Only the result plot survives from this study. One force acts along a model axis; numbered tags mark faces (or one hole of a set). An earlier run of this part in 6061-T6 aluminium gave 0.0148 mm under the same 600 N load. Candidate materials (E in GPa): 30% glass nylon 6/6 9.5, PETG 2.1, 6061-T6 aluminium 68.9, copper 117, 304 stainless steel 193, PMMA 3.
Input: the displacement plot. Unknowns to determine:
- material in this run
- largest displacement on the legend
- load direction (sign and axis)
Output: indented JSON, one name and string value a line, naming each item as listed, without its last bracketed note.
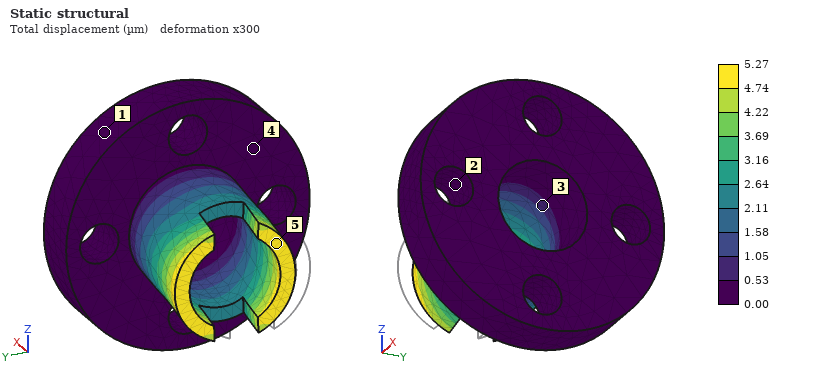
{
  "material in this run": "304 stainless steel",
  "largest displacement on the legend": "5.27 µm",
  "load direction": "+Y"
}
